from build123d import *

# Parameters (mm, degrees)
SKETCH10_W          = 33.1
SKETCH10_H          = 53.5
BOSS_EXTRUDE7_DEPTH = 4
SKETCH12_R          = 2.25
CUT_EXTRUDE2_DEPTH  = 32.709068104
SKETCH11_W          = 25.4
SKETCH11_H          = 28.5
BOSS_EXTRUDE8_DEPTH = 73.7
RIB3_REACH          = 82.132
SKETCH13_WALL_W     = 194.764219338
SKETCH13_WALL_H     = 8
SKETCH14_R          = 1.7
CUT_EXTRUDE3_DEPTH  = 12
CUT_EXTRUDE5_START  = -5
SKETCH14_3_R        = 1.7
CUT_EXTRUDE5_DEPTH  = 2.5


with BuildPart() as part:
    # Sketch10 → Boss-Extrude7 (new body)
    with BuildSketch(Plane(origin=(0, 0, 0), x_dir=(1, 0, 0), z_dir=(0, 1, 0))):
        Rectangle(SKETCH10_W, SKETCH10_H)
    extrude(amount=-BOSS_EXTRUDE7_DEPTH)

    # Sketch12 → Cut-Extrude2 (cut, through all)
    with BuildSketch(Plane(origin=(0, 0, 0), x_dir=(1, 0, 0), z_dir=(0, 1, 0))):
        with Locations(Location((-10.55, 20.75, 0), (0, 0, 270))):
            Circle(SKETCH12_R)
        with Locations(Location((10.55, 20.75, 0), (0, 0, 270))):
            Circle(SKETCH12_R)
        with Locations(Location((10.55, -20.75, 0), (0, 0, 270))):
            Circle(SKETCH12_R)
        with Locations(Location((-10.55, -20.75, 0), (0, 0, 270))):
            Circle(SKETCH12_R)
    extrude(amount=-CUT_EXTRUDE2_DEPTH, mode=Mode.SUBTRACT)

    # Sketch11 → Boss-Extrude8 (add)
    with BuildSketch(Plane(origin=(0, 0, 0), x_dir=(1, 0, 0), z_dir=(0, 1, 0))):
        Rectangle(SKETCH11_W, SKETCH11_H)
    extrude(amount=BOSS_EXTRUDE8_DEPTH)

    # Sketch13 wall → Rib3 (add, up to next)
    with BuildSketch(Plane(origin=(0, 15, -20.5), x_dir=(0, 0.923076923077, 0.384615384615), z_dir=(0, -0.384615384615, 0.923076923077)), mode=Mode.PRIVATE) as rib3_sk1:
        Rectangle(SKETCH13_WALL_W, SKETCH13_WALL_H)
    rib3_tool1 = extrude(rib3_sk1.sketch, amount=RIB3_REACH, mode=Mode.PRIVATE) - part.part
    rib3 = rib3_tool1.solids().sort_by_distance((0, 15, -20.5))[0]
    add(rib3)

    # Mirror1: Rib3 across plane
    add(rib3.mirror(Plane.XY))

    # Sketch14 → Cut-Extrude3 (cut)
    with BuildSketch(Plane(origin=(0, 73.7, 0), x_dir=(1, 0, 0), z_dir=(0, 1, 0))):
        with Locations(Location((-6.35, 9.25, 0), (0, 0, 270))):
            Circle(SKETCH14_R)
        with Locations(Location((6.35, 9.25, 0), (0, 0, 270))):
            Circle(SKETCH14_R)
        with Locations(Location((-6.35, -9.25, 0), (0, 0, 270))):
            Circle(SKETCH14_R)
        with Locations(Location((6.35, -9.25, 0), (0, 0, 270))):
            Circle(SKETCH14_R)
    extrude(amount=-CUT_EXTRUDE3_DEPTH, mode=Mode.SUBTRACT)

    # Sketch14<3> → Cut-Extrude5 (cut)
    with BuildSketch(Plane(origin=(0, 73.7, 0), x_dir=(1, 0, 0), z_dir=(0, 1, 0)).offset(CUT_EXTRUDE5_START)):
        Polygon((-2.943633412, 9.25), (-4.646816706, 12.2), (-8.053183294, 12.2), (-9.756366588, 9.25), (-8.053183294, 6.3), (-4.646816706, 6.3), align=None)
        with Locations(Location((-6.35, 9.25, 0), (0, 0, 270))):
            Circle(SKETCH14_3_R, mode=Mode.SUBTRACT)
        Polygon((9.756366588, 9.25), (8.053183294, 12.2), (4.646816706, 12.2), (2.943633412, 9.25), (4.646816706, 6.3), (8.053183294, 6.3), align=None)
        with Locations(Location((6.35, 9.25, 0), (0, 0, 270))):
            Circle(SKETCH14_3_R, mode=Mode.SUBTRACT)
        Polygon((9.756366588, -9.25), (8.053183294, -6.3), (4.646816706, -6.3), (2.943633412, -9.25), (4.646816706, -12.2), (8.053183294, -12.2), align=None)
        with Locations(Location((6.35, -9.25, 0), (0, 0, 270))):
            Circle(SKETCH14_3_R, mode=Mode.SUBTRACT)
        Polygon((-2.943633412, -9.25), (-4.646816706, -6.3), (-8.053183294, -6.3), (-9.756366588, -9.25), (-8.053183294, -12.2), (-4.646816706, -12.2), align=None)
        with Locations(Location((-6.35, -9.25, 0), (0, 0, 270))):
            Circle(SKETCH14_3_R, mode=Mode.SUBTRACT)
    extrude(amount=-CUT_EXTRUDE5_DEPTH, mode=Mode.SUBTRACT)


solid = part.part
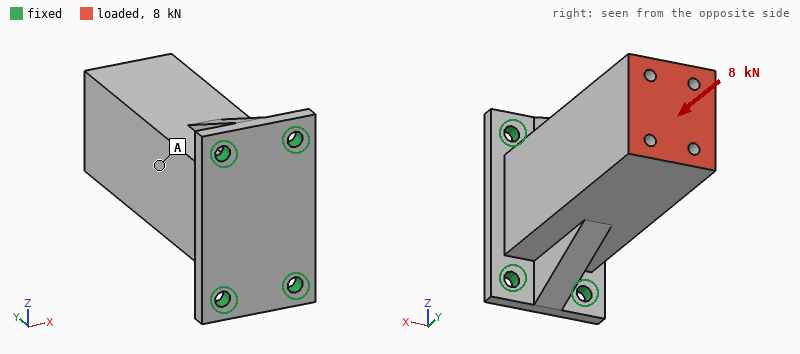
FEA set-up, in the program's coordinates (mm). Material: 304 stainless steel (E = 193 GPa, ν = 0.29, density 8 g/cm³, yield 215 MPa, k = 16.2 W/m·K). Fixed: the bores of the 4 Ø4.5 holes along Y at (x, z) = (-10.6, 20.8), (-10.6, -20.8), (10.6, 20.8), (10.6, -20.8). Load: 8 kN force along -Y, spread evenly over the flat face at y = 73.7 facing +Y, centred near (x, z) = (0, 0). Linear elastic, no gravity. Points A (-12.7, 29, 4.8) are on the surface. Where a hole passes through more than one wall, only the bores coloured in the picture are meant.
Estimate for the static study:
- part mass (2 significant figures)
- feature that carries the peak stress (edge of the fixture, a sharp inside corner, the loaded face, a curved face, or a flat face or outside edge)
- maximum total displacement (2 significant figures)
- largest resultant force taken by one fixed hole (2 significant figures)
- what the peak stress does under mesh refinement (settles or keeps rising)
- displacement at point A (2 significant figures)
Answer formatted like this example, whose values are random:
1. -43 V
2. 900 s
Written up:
1. 500 g
2. edge of the fixture
3. 11 µm
4. 2.2 kN
5. keeps rising
6. 8.0 µm
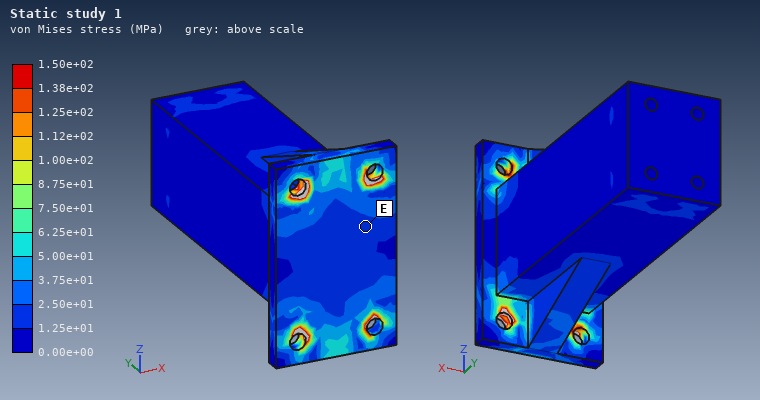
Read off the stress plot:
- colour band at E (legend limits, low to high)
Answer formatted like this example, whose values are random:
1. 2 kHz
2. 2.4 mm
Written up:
1. 1.25e+01 to 2.50e+01 MPa
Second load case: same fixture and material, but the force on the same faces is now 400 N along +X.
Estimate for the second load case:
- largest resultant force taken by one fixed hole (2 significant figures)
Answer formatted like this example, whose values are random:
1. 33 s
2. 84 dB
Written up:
1. 780 N
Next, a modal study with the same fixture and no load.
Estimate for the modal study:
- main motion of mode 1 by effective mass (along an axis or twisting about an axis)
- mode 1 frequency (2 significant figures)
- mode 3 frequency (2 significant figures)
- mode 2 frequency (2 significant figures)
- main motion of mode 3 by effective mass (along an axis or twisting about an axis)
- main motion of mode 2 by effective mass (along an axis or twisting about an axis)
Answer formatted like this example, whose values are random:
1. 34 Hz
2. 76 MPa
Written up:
1. along X
2. 1500 Hz
3. 7400 Hz
4. 3000 Hz
5. along Y
6. along Z
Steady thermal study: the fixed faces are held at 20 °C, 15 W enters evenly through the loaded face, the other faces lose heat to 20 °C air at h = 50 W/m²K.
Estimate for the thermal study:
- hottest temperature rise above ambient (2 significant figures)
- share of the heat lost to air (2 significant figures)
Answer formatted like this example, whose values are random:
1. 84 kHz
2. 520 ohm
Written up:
1. 53 K
2. 79 %
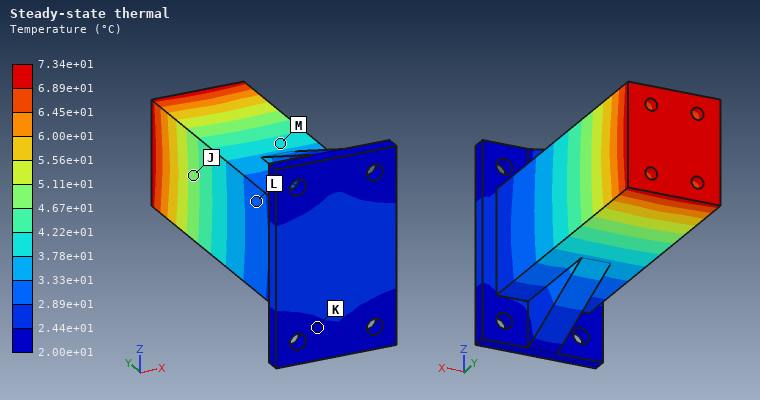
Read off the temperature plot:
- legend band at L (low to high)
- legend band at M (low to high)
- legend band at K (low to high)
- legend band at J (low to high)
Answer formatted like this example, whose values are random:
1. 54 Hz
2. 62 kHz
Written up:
1. 2.89e+01 to 3.33e+01 °C
2. 3.78e+01 to 4.22e+01 °C
3. 2.00e+01 to 2.44e+01 °C
4. 4.67e+01 to 5.11e+01 °C
